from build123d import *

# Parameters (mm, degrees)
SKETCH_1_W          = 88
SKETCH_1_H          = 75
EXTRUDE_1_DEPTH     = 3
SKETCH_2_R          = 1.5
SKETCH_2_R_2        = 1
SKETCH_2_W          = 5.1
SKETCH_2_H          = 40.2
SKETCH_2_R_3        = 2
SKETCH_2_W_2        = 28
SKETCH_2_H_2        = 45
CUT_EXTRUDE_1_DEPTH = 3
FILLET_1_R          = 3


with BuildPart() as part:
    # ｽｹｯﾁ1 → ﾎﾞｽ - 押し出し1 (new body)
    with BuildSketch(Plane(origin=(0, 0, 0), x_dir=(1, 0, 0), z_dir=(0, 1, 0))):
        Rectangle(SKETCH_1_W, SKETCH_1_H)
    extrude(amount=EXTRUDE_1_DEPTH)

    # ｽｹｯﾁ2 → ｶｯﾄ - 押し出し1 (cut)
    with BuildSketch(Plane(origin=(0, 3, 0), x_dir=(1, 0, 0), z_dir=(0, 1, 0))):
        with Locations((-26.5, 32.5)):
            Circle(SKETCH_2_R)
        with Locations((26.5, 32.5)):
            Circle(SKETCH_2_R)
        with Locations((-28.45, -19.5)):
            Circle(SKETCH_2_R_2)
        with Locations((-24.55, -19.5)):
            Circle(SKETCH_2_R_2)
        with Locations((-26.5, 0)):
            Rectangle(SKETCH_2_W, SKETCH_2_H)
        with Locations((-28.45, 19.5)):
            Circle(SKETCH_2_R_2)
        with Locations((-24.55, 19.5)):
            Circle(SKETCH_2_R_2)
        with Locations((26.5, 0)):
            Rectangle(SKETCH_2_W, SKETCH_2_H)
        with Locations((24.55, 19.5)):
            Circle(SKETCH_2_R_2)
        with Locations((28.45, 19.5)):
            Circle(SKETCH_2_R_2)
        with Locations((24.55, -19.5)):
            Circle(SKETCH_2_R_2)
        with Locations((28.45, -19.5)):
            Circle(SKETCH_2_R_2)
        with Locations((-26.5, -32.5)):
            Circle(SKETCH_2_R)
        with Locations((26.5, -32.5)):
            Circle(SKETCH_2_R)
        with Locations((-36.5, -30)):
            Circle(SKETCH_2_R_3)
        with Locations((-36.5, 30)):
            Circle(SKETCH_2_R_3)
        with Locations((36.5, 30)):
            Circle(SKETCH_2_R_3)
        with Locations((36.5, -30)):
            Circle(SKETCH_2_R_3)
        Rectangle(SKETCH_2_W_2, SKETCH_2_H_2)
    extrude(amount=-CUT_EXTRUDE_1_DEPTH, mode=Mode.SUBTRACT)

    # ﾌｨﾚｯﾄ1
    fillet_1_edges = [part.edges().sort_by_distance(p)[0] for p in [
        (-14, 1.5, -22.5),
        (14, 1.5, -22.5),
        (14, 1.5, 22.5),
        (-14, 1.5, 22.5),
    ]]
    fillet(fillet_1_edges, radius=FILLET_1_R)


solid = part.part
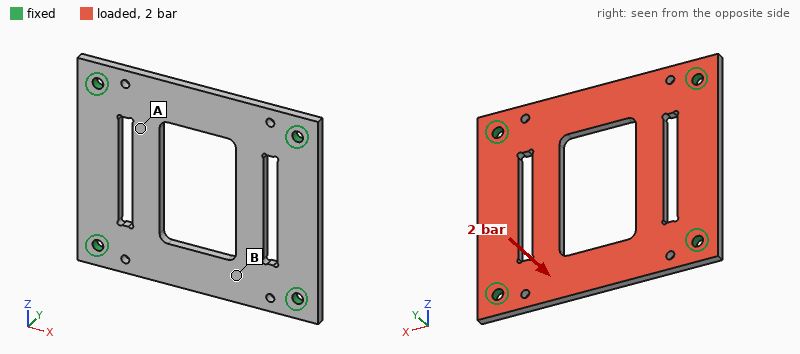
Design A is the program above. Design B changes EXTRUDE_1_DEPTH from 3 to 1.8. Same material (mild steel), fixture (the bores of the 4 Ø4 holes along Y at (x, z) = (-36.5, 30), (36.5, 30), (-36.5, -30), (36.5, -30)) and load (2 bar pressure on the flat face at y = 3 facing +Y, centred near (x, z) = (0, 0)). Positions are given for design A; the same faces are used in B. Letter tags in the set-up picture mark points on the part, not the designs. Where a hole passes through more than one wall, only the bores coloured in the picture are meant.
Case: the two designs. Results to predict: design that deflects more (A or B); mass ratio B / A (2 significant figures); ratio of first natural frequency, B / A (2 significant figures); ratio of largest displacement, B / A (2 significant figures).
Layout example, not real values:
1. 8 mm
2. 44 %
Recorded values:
1. B
2. 0.60
3. 0.62
4. 4.3
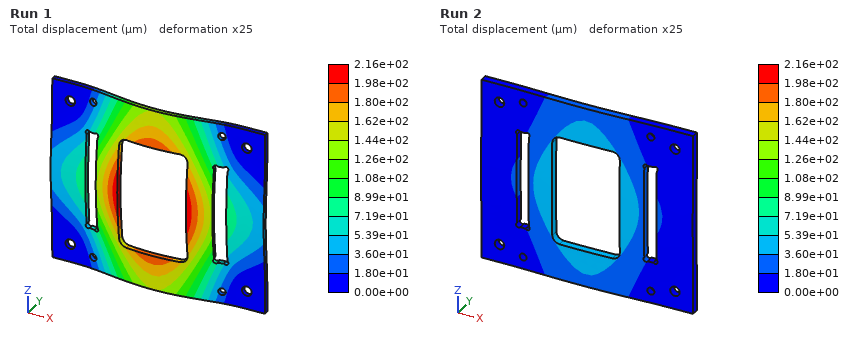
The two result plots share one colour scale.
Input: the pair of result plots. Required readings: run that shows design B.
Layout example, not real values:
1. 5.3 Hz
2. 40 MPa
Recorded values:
1. Run 1
